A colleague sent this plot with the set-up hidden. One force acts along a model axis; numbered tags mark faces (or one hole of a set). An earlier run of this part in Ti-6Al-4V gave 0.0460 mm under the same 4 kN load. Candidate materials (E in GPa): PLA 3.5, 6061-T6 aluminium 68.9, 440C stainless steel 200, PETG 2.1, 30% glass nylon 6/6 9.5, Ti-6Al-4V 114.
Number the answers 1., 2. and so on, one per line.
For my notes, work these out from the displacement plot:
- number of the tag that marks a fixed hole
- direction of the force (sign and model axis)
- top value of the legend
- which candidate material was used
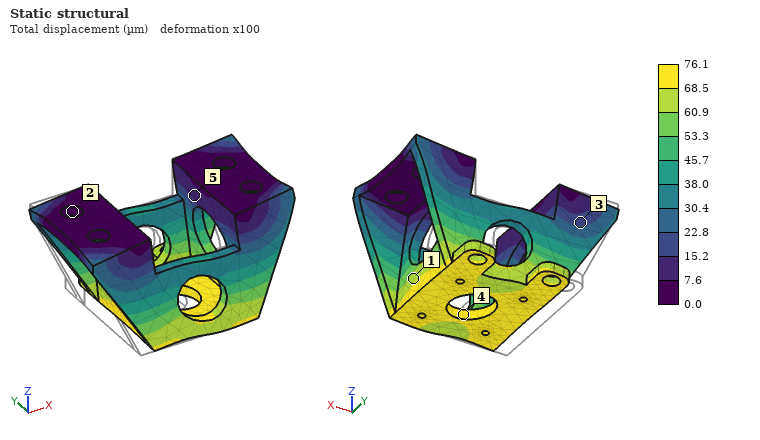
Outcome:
1. 2
2. +X
3. 76.1 µm
4. 6061-T6 aluminium
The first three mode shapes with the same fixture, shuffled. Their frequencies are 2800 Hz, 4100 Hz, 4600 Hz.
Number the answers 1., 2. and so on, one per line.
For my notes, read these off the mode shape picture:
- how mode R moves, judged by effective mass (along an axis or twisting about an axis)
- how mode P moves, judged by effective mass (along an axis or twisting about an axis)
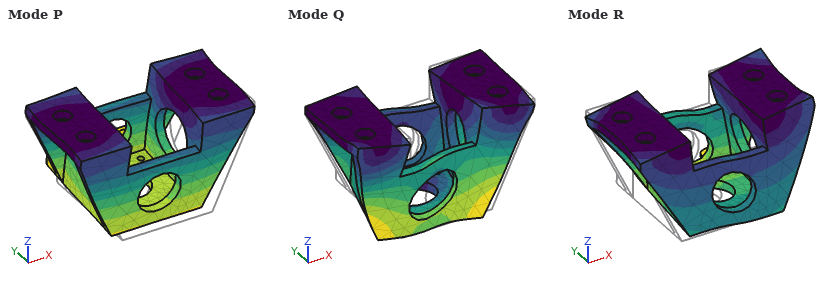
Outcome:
1. along X
2. along Y
